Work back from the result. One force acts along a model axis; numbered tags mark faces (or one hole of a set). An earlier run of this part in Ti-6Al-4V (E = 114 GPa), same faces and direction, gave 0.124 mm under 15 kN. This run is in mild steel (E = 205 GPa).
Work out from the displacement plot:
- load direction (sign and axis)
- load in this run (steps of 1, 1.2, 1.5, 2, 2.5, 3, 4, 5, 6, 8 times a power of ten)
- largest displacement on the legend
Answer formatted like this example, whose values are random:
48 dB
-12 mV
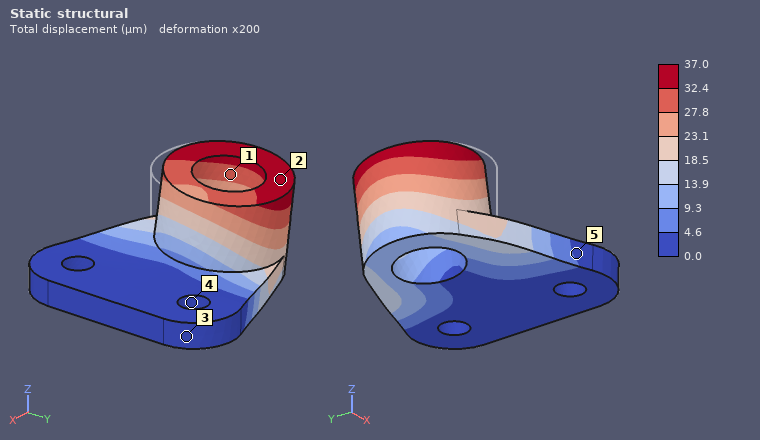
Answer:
+Y
8 kN
37.0 µm
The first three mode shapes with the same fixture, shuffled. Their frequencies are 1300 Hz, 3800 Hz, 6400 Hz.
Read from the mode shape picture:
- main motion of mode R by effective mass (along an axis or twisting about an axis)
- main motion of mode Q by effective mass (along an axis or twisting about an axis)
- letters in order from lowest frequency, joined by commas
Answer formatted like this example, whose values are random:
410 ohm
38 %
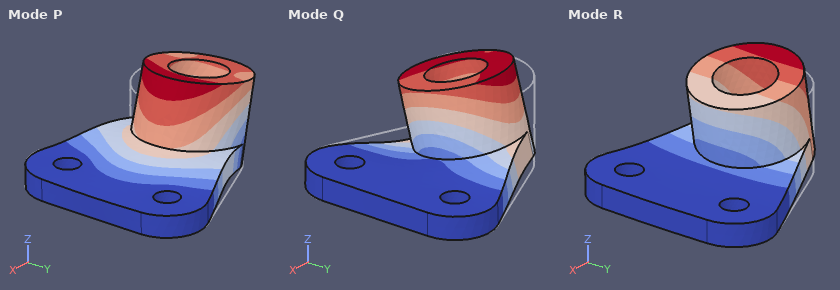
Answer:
along Z
along Y
R, Q, P
